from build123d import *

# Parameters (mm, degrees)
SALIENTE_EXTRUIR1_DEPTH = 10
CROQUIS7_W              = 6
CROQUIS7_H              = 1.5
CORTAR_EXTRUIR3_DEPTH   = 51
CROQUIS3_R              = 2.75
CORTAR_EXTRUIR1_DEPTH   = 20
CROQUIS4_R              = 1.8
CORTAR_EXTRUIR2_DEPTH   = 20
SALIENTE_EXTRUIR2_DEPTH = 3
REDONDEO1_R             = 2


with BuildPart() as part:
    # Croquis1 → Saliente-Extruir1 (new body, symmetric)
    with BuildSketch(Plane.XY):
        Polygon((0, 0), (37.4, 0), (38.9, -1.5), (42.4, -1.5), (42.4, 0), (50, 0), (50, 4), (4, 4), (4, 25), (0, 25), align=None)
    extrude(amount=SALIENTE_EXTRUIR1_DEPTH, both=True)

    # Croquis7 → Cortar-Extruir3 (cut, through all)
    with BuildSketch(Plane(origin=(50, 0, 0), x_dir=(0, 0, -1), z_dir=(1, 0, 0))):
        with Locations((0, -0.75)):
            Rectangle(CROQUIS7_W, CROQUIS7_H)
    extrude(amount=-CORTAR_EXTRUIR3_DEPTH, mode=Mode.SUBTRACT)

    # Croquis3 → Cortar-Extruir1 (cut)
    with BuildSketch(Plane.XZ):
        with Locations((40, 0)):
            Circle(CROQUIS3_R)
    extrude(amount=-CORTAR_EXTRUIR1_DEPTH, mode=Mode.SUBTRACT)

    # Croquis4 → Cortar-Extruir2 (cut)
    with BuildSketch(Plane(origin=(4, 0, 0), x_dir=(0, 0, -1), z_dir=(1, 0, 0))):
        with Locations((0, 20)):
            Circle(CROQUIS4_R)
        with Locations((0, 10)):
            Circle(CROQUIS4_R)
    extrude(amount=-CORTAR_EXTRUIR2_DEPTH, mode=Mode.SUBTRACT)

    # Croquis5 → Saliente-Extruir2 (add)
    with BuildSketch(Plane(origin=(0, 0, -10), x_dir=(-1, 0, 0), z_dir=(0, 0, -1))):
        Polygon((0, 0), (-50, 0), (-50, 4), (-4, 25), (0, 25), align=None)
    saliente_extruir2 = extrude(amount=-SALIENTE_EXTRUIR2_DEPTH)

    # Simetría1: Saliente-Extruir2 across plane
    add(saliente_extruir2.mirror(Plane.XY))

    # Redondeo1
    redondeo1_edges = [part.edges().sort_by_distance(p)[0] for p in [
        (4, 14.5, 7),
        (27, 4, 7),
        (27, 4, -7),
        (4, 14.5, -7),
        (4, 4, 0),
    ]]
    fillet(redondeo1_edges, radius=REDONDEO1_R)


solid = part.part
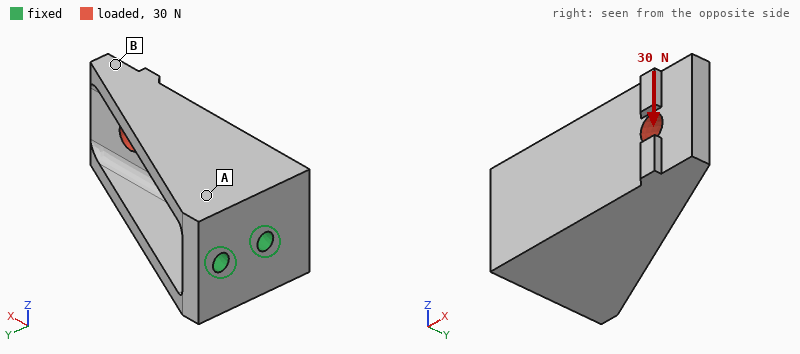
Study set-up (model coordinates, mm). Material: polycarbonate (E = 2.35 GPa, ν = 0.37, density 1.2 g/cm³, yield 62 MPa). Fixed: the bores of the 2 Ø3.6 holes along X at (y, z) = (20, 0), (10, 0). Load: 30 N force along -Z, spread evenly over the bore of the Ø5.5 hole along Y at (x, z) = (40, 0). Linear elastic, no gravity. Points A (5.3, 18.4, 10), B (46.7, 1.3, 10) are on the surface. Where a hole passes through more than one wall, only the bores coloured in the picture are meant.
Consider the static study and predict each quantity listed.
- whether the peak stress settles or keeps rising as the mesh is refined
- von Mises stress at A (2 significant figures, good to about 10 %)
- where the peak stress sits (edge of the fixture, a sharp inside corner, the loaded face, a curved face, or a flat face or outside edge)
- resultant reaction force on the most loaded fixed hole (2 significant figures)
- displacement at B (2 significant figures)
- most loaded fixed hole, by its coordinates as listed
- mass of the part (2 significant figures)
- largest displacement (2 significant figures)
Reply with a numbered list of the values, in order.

1. keeps rising
2. 3.1 MPa
3. edge of the fixture
4. 44 N
5. 0.48 mm
6. (10, 0)
7. 10 g
8. 0.54 mm
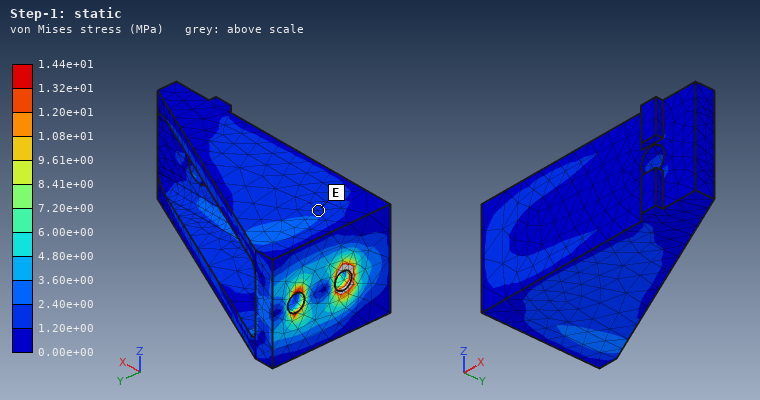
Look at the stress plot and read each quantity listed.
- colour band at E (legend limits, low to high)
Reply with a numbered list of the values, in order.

1. 1.20e+00 to 2.40e+00 MPa
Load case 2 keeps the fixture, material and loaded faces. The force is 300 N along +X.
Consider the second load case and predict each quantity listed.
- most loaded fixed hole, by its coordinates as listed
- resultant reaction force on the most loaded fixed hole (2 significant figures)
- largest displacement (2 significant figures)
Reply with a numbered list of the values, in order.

1. (10, 0)
2. 410 N
3. 0.62 mm
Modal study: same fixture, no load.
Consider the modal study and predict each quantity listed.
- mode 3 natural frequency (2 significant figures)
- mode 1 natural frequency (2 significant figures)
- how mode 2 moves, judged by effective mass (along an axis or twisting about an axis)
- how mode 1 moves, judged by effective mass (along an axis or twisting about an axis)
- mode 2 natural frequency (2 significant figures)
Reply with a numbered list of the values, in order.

1. 2500 Hz
2. 690 Hz
3. along Y
4. along Z
5. 1100 Hz
